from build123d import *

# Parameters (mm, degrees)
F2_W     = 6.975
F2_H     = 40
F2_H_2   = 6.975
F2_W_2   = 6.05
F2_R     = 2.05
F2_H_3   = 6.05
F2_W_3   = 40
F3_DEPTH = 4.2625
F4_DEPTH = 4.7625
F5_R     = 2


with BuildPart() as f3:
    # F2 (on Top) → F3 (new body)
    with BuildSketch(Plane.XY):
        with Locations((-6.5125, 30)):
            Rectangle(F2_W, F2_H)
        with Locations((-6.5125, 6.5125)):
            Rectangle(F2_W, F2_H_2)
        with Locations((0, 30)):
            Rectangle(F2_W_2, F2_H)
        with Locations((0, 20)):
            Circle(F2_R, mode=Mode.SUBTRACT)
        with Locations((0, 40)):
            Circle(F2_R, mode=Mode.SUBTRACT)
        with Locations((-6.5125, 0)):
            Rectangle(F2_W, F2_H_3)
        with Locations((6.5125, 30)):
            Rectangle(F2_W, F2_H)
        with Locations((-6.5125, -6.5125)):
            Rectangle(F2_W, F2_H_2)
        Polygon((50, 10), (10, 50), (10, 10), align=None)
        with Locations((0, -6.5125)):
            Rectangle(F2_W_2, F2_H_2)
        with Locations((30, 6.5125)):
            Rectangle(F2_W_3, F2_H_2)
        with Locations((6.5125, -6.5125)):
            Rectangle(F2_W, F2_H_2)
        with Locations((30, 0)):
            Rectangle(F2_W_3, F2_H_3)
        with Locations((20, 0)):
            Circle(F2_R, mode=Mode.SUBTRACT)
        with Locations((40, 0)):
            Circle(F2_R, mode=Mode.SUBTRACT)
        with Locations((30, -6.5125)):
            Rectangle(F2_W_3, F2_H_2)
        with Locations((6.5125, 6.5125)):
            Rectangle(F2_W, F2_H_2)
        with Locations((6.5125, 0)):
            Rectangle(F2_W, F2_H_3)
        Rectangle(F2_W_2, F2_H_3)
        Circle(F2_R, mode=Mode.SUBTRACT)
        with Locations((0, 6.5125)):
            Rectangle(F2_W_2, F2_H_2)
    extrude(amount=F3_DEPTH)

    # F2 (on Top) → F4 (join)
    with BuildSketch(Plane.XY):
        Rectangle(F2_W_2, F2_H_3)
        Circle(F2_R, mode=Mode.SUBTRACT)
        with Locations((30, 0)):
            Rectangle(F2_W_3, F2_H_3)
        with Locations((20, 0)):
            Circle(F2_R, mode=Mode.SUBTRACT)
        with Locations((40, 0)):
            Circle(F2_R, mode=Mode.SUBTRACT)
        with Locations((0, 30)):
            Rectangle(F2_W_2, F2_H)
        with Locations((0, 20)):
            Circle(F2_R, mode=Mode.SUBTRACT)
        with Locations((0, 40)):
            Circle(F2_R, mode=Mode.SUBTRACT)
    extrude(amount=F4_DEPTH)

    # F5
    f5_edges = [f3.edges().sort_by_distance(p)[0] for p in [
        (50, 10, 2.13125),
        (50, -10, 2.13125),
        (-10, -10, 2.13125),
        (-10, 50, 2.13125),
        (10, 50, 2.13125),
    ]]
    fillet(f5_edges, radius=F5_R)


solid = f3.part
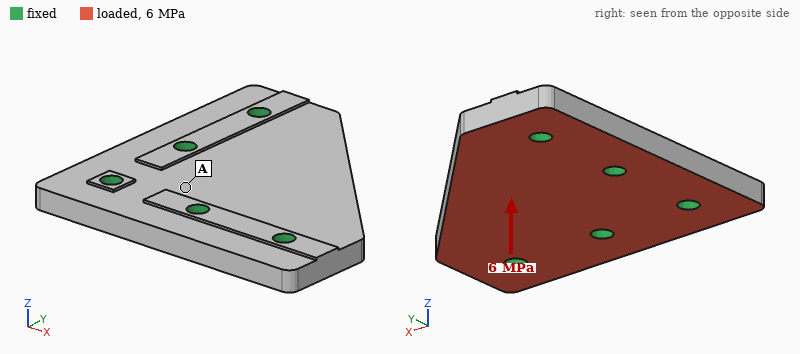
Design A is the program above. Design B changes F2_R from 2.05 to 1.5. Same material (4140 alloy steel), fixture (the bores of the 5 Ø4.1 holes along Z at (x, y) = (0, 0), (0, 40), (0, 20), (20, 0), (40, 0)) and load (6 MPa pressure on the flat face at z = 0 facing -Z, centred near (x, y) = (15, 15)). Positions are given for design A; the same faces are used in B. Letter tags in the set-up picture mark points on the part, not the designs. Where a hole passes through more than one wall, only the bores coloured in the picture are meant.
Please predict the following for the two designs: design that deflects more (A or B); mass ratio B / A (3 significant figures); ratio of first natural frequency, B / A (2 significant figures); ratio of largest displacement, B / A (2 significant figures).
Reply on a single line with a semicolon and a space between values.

B; 1.01; 0.94; 1.1
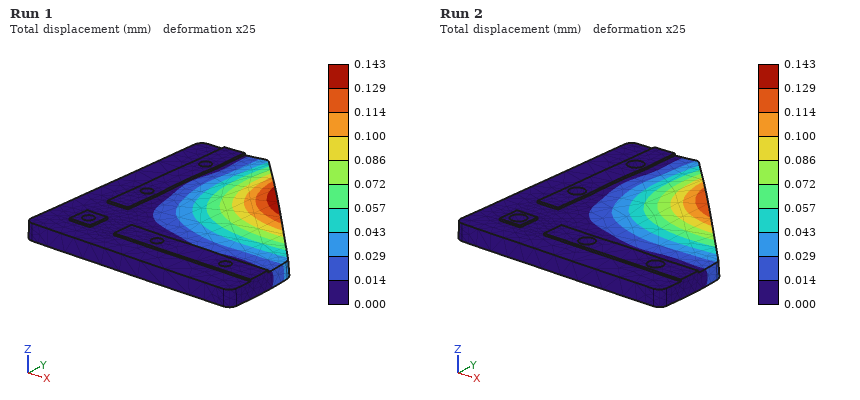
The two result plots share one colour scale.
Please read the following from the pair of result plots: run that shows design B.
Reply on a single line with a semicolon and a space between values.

Run 1
